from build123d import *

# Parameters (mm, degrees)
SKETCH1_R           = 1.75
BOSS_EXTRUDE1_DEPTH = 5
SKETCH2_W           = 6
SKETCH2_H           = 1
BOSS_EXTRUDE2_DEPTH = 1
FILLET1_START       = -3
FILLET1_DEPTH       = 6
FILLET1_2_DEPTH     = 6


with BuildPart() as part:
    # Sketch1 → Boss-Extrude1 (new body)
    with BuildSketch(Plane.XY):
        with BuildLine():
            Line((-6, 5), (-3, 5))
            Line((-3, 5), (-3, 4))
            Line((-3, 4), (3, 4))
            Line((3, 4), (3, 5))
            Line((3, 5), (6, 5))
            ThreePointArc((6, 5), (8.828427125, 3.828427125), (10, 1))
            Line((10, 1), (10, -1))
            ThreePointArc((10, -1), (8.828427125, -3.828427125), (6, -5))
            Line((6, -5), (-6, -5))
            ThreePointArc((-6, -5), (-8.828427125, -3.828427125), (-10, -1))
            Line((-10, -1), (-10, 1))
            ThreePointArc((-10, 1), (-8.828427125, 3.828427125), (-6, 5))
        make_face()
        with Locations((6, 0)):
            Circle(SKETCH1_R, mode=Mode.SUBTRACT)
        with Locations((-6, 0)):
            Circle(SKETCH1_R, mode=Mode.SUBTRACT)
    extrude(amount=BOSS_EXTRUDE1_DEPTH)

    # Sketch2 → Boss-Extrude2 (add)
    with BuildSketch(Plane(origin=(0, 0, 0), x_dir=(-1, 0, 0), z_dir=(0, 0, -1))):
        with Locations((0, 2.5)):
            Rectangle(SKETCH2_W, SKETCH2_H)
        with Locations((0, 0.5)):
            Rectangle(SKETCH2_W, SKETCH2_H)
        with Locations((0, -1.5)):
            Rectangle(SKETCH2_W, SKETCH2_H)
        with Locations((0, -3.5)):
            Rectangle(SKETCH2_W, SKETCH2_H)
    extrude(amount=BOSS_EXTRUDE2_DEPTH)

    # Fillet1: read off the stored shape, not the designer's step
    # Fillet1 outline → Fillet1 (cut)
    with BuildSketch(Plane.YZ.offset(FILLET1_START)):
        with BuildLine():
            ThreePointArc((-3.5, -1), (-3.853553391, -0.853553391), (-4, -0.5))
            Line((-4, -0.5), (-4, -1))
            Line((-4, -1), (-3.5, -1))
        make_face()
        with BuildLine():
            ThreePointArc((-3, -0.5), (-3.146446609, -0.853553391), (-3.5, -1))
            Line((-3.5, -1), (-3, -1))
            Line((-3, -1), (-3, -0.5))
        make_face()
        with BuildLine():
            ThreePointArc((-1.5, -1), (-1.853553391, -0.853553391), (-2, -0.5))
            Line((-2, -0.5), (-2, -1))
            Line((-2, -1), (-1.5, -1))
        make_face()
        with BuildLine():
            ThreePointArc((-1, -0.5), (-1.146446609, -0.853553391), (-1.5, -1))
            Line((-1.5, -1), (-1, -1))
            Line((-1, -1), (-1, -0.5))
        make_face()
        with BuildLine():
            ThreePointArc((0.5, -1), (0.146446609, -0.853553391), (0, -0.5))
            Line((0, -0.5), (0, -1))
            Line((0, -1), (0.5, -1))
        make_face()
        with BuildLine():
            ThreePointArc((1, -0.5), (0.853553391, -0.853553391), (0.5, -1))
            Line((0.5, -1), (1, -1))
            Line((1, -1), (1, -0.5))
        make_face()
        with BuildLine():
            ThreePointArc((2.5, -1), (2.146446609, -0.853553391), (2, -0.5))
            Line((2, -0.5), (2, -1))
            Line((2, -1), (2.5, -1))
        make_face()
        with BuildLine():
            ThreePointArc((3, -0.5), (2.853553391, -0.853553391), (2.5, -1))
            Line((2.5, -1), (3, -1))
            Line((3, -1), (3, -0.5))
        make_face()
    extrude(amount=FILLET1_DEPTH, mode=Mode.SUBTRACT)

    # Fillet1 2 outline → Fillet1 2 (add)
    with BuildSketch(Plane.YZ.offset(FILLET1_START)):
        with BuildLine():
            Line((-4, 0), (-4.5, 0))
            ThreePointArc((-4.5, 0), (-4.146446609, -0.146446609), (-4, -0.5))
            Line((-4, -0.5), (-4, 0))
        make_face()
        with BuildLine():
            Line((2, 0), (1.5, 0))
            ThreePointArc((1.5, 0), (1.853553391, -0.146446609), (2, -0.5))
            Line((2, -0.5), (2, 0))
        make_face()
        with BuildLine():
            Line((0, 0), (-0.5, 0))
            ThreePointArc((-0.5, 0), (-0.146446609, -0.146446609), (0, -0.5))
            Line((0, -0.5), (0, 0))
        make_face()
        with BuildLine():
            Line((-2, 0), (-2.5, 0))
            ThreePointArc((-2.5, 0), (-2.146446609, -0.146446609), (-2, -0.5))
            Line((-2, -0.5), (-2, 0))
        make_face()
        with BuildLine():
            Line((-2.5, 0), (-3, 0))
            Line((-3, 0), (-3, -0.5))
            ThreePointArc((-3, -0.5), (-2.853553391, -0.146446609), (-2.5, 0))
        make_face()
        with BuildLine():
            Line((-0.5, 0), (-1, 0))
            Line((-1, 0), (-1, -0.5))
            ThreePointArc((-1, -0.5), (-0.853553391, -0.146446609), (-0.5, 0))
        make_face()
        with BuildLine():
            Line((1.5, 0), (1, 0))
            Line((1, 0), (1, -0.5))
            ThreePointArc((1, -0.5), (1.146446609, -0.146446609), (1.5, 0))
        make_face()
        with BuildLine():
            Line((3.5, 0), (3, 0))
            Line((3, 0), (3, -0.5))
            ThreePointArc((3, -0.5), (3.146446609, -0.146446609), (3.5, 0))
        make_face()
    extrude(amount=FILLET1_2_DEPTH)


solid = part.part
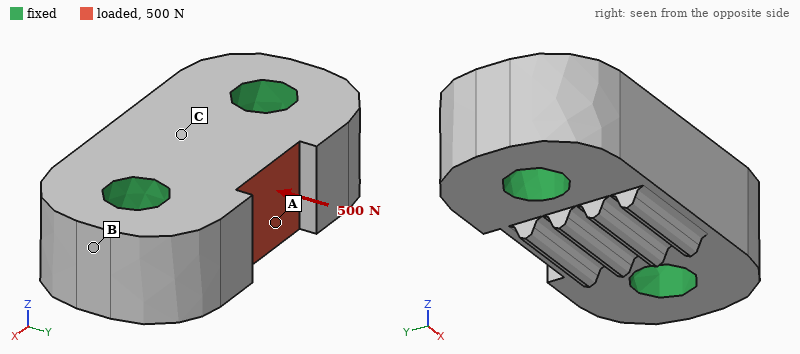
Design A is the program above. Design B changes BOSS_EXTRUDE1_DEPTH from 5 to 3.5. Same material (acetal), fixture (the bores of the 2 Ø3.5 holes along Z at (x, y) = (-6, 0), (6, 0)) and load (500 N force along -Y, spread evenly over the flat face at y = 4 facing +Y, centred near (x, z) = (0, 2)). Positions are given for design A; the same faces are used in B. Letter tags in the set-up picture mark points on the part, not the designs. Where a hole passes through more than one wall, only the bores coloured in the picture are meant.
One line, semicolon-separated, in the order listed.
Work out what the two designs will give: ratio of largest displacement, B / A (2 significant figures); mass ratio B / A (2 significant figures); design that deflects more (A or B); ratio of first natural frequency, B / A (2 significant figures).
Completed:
1.4; 0.71; B; 0.87
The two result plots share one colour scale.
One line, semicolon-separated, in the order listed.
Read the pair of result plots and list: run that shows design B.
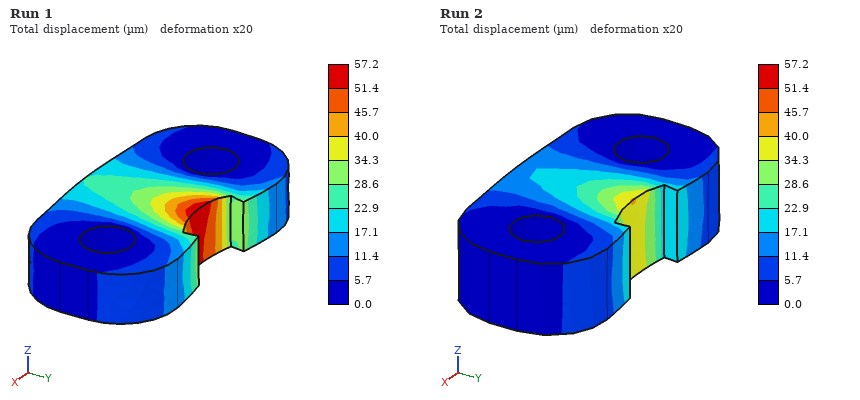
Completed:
Run 1
